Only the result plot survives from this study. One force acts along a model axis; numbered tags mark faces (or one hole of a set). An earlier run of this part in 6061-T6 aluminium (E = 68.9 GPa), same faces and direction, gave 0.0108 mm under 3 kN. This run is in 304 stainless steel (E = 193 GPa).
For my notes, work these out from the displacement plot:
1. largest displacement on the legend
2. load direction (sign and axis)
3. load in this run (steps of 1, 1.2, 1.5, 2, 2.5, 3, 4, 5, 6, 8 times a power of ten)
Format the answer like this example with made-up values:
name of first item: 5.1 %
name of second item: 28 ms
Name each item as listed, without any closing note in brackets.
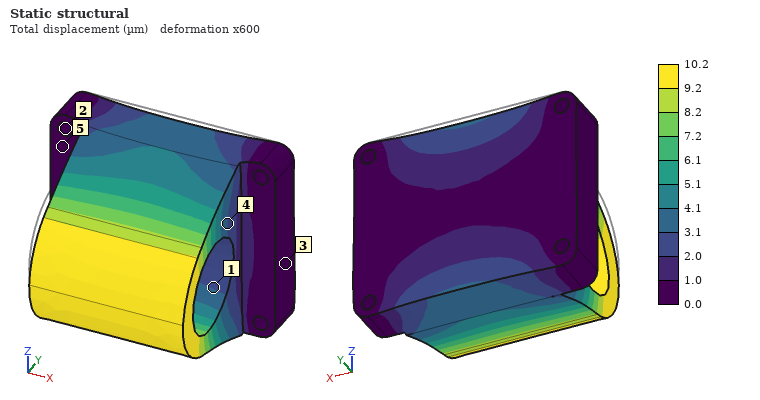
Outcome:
largest displacement on the legend: 10.2 µm
load direction: -Z
load in this run: 8 kN
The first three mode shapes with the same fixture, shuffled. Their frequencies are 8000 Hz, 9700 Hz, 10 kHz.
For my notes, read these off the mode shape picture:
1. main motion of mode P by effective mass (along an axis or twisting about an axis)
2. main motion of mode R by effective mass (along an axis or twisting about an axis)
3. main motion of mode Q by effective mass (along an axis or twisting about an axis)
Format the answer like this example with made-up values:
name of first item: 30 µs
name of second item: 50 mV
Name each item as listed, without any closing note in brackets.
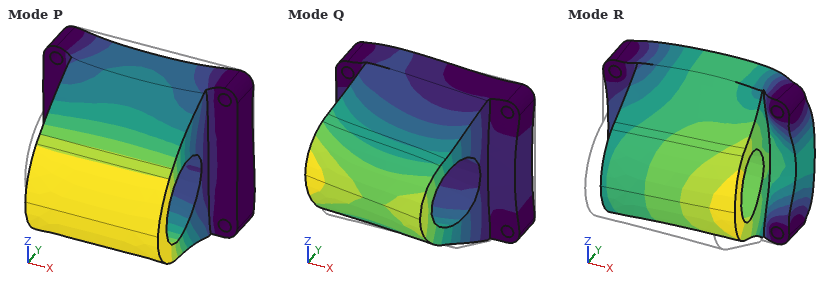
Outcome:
main motion of mode P by effective mass: along Z
main motion of mode R by effective mass: along Y
main motion of mode Q by effective mass: along X
